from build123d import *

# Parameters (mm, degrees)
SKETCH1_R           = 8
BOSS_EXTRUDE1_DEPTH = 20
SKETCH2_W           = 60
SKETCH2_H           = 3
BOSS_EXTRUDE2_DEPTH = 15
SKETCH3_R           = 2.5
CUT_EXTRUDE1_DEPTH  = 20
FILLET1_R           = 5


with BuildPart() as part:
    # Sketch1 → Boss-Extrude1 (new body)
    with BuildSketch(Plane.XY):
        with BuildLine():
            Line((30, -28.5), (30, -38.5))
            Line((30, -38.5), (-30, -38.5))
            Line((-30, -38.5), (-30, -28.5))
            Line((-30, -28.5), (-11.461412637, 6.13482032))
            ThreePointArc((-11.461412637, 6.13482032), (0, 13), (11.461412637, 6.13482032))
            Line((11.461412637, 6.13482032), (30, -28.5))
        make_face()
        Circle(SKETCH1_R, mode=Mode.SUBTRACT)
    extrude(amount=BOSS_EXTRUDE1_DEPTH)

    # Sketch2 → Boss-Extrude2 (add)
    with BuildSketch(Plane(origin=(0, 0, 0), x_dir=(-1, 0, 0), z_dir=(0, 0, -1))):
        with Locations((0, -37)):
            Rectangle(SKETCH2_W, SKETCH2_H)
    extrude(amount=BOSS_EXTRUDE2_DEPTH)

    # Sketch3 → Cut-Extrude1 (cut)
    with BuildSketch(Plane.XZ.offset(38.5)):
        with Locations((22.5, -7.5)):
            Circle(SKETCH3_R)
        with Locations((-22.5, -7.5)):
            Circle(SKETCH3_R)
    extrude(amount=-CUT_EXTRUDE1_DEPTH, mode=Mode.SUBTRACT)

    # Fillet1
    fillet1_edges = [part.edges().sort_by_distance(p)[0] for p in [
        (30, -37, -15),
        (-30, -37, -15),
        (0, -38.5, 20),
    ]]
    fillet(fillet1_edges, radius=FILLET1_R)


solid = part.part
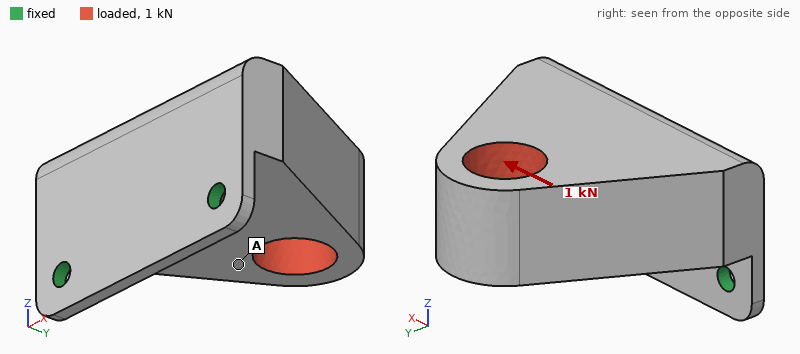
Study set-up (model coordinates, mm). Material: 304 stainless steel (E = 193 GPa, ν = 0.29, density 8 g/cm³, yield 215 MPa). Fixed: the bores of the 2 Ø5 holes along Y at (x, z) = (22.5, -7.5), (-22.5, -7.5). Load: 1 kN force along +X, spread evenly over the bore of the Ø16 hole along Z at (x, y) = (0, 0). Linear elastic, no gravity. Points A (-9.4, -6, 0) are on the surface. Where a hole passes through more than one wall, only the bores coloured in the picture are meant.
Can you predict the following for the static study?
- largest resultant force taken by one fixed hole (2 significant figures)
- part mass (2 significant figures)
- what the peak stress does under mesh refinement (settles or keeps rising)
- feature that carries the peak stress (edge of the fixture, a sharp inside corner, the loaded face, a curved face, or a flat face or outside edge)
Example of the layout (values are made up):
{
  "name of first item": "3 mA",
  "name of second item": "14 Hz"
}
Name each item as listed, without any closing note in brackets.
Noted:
{
  "largest resultant force taken by one fixed hole": "1.0 kN",
  "part mass": "330 g",
  "what the peak stress does under mesh refinement": "keeps rising",
  "feature that carries the peak stress": "edge of the fixture"
}
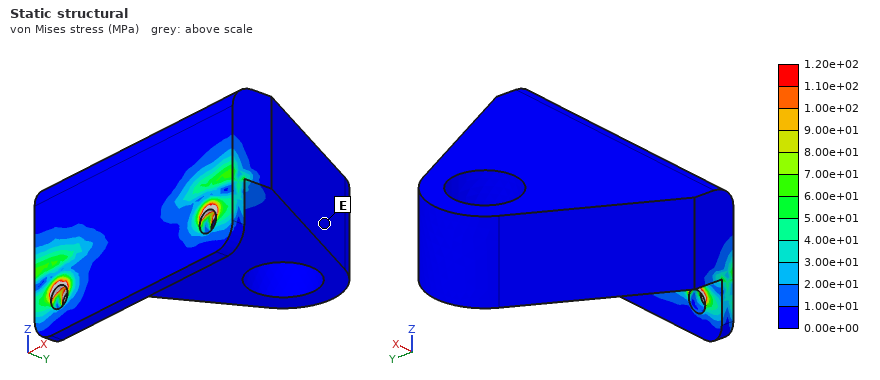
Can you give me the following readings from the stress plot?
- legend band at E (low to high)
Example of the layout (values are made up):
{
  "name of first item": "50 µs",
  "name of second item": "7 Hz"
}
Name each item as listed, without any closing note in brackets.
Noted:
{
  "legend band at E": "0.00e+00 to 1.00e+01 MPa"
}
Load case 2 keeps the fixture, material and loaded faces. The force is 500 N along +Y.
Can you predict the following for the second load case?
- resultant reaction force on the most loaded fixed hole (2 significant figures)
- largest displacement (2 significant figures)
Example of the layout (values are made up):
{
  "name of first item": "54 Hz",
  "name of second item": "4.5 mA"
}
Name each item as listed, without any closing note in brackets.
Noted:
{
  "resultant reaction force on the most loaded fixed hole": "250 N",
  "largest displacement": "0.14 mm"
}
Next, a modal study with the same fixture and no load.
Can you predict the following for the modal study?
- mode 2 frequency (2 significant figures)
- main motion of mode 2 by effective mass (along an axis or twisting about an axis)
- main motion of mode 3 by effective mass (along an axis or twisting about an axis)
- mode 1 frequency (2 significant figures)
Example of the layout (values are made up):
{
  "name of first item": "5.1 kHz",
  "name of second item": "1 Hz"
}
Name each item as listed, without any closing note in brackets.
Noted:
{
  "mode 2 frequency": "3400 Hz",
  "main motion of mode 2 by effective mass": "along X",
  "main motion of mode 3 by effective mass": "along Y",
  "mode 1 frequency": "570 Hz"
}
